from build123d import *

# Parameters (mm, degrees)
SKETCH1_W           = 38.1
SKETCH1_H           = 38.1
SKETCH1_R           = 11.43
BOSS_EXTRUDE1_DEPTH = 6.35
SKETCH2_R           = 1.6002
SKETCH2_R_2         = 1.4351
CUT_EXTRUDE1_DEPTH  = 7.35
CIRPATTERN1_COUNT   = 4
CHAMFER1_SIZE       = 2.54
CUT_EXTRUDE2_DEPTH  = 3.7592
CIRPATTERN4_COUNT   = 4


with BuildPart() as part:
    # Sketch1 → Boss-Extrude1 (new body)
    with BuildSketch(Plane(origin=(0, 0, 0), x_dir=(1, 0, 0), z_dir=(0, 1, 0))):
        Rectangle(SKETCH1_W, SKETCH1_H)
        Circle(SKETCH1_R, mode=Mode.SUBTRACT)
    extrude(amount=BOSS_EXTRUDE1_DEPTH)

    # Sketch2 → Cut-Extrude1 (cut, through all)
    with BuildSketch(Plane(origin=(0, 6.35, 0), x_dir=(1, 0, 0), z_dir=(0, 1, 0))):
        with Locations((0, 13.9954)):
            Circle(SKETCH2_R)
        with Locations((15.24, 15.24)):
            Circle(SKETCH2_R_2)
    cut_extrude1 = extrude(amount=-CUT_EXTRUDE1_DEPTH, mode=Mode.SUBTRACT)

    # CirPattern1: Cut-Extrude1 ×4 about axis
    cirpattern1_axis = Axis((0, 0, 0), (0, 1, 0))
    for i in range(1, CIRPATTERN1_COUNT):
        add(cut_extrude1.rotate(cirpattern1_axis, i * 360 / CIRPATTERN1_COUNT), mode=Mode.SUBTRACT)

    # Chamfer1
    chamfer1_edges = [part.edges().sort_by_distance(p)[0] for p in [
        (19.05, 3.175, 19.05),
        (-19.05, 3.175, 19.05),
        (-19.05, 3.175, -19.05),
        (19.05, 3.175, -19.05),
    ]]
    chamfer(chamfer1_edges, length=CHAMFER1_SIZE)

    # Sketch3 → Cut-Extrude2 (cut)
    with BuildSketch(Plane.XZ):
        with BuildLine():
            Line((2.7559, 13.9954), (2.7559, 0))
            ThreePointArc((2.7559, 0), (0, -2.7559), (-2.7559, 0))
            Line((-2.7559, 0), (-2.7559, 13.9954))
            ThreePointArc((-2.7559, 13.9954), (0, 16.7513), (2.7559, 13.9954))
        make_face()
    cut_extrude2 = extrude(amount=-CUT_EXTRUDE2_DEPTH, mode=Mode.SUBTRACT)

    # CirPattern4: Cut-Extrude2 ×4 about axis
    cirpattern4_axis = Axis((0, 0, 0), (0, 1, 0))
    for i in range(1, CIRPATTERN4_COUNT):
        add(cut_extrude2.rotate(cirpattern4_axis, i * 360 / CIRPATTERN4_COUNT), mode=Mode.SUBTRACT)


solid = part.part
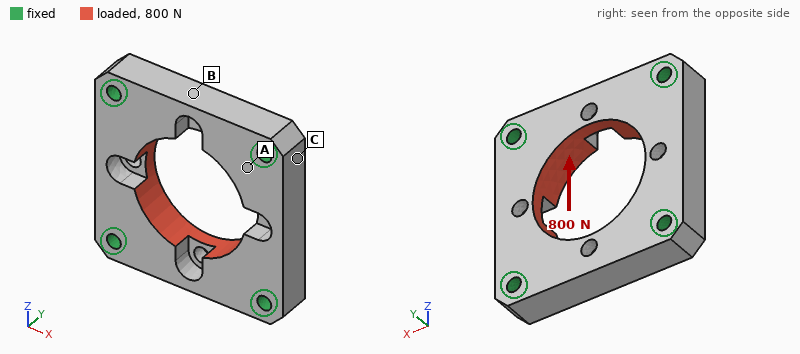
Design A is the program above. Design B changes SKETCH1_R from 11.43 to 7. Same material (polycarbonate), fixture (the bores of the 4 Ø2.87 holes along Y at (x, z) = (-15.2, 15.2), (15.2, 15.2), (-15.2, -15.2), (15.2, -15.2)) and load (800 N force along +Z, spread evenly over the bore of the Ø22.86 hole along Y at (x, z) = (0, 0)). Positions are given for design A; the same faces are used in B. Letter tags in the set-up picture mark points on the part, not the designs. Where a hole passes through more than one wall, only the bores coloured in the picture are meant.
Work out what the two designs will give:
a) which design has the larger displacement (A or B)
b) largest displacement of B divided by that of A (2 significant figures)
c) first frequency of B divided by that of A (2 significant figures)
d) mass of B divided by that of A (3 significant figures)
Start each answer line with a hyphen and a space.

- A
- 0.90
- 0.90
- 1.21
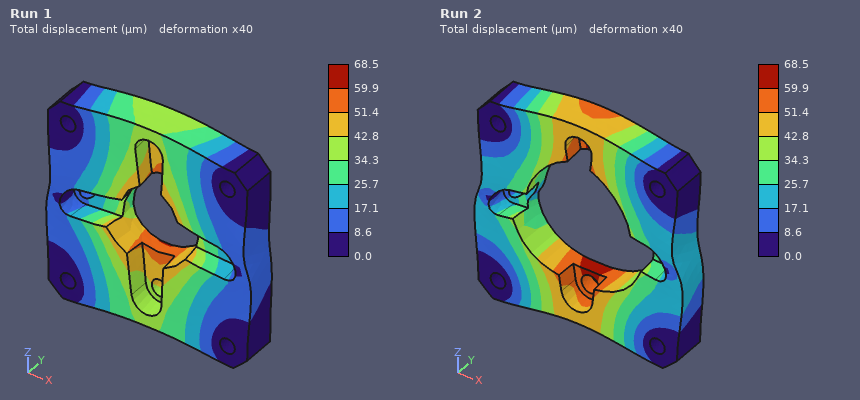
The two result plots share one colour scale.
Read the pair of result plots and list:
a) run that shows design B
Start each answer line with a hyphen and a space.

- Run 1
